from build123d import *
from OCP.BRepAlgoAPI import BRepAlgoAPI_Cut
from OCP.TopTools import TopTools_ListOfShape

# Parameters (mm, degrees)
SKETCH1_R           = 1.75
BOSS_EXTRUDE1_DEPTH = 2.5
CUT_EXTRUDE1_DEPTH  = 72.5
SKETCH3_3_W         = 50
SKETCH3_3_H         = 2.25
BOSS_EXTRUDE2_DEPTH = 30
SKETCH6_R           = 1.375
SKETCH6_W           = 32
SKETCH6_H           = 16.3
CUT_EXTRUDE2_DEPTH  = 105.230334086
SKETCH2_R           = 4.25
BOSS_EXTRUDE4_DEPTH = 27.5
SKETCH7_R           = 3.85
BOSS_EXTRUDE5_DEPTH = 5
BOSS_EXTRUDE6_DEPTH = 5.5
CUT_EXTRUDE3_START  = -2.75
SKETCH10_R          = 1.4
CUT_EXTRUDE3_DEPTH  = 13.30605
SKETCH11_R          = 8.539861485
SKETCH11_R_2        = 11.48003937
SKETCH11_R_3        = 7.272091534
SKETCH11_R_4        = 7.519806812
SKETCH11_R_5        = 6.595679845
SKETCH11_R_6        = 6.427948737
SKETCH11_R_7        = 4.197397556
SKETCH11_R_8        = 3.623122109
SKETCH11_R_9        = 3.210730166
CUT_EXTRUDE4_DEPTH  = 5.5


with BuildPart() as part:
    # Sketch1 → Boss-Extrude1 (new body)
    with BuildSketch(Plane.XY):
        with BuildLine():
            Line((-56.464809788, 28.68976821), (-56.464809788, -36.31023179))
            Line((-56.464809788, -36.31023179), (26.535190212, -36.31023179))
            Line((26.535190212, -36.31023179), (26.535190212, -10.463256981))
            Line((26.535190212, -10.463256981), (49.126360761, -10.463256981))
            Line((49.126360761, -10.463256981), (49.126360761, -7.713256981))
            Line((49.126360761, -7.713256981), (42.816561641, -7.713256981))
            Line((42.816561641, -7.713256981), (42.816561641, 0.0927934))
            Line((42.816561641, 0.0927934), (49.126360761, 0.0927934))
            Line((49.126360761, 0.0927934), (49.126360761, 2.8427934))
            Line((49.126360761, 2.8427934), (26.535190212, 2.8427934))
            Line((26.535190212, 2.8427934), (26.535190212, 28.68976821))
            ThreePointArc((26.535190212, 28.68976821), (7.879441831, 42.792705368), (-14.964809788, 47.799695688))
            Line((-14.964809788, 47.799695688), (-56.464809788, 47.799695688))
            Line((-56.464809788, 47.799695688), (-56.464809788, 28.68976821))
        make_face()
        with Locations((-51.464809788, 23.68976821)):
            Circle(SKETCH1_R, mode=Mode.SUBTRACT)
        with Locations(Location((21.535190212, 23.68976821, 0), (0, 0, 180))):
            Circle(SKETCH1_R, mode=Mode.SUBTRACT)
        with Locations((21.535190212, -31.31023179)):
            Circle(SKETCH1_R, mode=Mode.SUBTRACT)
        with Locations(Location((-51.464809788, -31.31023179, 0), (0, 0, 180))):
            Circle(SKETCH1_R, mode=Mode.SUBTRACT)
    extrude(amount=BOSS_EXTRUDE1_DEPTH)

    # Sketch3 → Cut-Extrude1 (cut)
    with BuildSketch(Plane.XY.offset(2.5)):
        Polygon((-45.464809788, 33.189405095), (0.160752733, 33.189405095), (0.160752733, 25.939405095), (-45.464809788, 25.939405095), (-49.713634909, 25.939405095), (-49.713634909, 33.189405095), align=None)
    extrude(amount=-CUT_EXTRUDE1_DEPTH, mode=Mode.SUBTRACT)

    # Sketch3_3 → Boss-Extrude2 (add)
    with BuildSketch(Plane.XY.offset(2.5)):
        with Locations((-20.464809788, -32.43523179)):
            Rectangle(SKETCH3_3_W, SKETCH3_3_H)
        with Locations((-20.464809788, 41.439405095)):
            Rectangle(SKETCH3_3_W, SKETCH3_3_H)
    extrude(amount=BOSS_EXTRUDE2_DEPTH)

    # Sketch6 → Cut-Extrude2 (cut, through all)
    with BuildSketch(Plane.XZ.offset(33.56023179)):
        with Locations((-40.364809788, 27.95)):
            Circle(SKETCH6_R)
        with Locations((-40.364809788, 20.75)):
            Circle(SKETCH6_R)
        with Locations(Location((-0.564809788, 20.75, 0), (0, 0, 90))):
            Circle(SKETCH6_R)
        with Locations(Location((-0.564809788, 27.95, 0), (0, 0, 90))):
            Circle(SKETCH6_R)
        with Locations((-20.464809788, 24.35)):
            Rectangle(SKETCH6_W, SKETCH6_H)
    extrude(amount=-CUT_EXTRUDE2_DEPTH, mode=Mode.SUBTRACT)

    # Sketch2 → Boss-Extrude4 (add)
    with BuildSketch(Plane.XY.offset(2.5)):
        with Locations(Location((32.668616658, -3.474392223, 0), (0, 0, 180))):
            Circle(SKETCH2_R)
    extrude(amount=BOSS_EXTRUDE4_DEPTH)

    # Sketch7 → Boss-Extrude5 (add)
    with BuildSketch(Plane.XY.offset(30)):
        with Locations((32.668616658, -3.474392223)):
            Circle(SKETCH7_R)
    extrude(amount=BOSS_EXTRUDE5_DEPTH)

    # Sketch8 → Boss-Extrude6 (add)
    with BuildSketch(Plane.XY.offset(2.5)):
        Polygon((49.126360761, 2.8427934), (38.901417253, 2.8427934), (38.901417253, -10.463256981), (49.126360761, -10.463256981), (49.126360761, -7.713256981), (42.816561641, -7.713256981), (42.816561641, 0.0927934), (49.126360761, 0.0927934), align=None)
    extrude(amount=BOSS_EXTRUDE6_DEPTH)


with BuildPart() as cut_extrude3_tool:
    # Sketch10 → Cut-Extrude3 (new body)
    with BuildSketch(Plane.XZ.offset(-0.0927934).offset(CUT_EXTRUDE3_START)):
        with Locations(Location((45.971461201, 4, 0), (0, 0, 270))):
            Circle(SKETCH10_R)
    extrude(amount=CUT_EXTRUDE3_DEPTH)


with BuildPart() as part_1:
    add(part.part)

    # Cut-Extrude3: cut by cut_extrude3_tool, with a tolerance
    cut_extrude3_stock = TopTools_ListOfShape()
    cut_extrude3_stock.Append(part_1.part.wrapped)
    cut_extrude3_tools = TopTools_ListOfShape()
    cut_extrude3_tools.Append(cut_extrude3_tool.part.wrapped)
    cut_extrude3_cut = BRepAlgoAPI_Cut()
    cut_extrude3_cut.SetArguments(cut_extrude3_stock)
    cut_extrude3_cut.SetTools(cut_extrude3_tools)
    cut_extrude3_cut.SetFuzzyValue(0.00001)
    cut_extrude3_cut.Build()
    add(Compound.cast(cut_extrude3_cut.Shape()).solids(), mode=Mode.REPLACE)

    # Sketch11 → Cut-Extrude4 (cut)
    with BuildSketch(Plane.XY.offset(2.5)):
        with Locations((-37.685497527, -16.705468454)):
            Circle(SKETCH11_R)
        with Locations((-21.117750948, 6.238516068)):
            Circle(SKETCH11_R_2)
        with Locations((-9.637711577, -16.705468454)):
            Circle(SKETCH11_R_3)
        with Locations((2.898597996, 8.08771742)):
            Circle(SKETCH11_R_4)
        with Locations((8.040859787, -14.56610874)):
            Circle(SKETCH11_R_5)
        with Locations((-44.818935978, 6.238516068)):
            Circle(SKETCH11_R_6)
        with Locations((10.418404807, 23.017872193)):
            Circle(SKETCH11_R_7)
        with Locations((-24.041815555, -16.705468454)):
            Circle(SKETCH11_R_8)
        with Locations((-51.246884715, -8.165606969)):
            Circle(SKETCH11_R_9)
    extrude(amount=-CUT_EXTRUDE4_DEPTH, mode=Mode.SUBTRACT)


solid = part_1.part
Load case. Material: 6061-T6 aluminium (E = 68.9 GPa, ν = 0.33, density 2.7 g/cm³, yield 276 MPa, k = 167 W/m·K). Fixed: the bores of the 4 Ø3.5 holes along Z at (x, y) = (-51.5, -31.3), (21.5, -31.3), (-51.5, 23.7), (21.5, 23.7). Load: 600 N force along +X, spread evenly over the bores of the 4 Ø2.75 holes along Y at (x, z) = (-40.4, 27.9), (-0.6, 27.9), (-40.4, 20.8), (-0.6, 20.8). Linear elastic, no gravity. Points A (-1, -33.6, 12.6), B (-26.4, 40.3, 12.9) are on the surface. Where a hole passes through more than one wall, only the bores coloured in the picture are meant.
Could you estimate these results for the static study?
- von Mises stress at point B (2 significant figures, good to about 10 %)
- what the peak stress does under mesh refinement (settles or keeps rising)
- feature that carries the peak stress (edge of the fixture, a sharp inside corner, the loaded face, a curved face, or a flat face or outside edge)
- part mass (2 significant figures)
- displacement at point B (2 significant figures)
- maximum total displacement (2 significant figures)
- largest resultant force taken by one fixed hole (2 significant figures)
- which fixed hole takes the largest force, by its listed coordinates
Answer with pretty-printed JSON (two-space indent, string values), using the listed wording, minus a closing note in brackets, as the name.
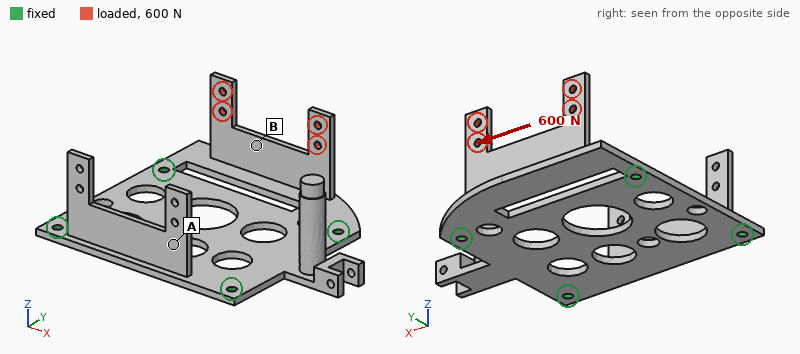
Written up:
{
  "von Mises stress at point B": "41 MPa",
  "what the peak stress does under mesh refinement": "keeps rising",
  "feature that carries the peak stress": "edge of the fixture",
  "part mass": "53 g",
  "displacement at point B": "0.15 mm",
  "maximum total displacement": "0.54 mm",
  "largest resultant force taken by one fixed hole": "480 N",
  "which fixed hole takes the largest force, by its listed coordinates": "(21.5, 23.7)"
}
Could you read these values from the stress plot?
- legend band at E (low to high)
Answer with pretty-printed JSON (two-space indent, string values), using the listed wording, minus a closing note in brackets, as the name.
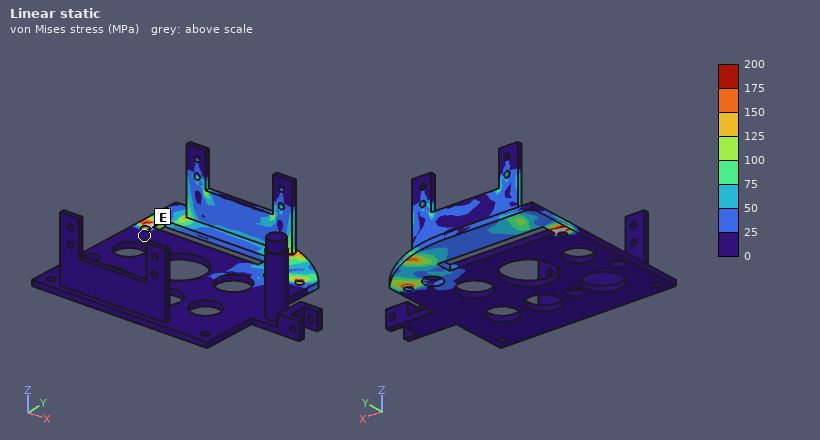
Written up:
{
  "legend band at E": "0 to 25 MPa"
}
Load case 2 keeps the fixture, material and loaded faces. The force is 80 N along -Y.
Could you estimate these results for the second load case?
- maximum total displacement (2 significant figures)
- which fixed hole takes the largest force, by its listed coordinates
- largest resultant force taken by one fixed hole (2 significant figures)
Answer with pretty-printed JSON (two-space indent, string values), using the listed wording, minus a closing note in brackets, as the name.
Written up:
{
  "maximum total displacement": "0.81 mm",
  "which fixed hole takes the largest force, by its listed coordinates": "(-51.5, 23.7)",
  "largest resultant force taken by one fixed hole": "40 N"
}
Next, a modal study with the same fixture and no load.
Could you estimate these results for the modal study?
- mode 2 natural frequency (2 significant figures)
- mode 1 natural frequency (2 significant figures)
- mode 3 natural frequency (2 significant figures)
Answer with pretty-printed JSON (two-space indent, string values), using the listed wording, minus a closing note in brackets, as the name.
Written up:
{
  "mode 2 natural frequency": "1000 Hz",
  "mode 1 natural frequency": "860 Hz",
  "mode 3 natural frequency": "1600 Hz"
}
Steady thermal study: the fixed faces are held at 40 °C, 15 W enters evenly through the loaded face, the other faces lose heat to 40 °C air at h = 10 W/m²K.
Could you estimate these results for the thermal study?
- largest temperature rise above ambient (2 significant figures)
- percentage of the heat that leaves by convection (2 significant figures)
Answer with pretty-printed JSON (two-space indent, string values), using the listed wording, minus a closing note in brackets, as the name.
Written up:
{
  "largest temperature rise above ambient": "75 K",
  "percentage of the heat that leaves by convection": "13 %"
}
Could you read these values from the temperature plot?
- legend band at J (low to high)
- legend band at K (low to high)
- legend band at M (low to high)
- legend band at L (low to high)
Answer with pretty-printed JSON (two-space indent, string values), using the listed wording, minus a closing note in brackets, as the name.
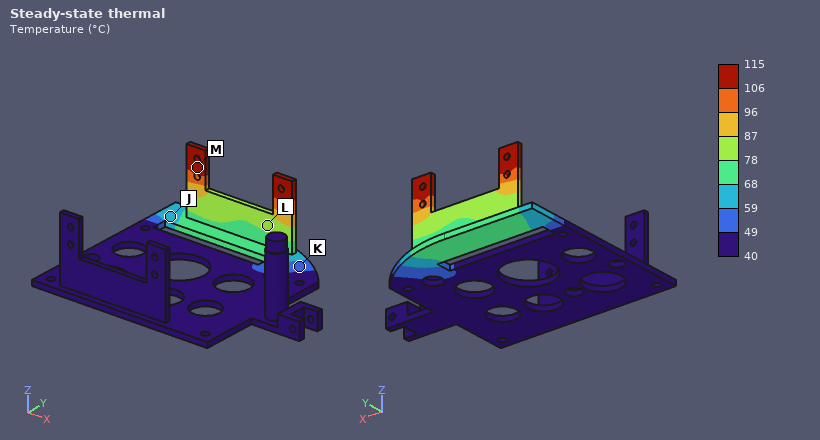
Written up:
{
  "legend band at J": "59 to 68 °C",
  "legend band at K": "49 to 59 °C",
  "legend band at M": "106 to 115 °C",
  "legend band at L": "78 to 87 °C"
}
